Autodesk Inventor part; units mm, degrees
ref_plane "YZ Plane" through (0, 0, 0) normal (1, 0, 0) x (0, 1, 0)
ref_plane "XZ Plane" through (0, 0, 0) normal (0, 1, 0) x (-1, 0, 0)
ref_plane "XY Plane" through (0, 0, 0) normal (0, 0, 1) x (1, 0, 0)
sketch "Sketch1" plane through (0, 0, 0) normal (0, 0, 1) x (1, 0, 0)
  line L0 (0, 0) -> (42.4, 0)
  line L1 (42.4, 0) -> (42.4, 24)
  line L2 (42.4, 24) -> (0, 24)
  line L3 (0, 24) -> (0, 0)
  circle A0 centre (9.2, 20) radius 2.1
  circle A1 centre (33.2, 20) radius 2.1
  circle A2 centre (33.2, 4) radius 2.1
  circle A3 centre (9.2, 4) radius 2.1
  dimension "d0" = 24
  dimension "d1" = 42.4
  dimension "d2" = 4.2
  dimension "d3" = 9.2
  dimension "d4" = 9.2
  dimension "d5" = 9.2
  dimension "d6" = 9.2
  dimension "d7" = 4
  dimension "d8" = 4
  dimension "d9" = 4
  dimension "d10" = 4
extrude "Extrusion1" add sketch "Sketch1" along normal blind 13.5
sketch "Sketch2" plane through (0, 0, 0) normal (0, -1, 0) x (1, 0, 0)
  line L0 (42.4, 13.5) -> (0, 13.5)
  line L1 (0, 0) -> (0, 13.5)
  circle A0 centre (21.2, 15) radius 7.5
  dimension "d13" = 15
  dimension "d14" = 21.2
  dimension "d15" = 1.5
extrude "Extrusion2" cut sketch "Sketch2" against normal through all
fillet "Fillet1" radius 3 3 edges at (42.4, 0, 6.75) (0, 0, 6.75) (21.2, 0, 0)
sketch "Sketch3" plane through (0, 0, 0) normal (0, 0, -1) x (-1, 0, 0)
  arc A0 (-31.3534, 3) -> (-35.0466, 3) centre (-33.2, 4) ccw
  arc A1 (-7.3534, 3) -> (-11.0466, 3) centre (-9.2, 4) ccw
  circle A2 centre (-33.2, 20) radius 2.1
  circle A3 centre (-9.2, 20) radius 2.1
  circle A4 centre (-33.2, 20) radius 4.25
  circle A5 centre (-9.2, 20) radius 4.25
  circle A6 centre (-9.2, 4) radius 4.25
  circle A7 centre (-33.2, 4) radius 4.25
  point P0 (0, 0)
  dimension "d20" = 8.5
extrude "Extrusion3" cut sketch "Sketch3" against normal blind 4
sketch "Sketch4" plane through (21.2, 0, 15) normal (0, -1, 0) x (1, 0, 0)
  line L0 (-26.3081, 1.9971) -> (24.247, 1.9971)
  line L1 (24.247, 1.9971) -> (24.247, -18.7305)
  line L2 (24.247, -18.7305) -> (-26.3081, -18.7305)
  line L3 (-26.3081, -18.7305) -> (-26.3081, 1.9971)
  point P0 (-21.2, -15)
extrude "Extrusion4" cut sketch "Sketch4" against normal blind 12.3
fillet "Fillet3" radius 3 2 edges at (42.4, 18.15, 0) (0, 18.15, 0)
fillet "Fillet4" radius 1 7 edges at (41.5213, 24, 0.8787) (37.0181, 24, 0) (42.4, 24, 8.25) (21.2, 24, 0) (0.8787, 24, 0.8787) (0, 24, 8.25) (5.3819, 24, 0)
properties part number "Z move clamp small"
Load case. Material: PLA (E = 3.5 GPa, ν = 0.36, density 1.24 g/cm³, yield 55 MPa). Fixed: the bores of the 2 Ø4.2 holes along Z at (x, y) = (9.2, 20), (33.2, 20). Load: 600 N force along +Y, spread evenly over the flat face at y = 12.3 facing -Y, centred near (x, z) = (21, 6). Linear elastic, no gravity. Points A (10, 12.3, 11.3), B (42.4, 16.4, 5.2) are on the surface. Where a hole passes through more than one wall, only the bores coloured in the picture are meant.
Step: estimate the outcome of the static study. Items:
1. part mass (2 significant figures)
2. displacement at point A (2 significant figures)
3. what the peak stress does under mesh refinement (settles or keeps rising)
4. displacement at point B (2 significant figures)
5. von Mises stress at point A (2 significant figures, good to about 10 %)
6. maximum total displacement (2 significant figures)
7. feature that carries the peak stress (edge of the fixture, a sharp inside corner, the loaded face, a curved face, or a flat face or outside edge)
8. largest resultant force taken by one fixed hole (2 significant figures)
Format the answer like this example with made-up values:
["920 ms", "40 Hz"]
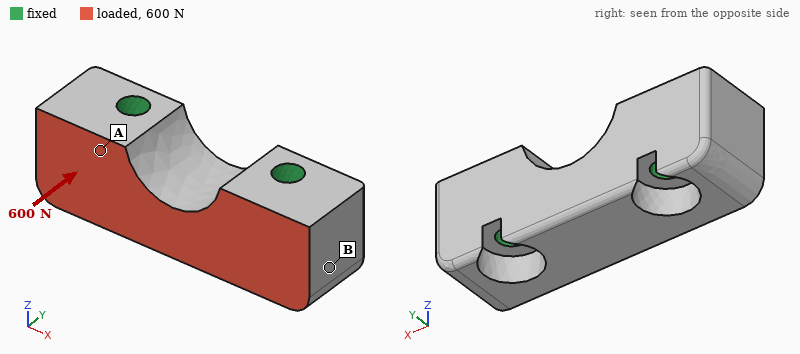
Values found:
["6.4 g", "5.3 µm", "keeps rising", "11 µm", "2.5 MPa", "22 µm", "edge of the fixture", "300 N"]
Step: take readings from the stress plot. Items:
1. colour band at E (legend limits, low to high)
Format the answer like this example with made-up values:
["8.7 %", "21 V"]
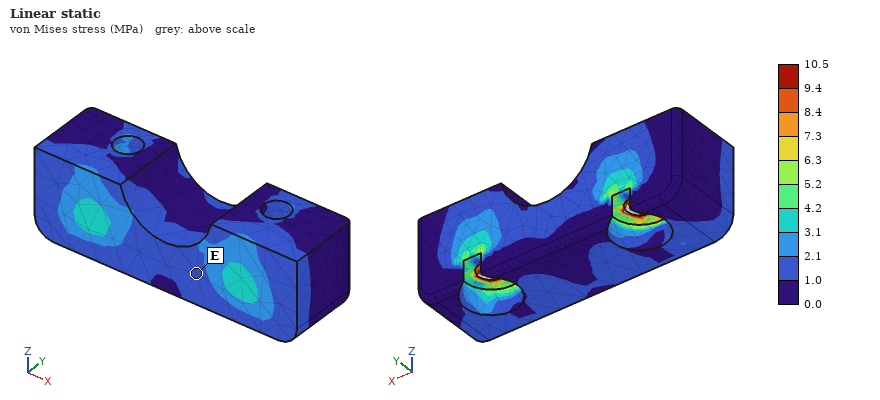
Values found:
["1.0 to 2.1 MPa"]
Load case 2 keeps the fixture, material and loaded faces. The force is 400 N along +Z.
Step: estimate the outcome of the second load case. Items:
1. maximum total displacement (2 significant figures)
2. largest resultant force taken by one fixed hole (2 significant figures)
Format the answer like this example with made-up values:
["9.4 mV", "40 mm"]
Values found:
["31 µm", "200 N"]
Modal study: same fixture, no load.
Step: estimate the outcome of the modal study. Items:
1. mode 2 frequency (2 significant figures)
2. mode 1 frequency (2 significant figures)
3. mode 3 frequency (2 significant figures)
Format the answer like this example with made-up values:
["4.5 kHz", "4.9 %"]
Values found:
["14 kHz", "12 kHz", "14 kHz"]
